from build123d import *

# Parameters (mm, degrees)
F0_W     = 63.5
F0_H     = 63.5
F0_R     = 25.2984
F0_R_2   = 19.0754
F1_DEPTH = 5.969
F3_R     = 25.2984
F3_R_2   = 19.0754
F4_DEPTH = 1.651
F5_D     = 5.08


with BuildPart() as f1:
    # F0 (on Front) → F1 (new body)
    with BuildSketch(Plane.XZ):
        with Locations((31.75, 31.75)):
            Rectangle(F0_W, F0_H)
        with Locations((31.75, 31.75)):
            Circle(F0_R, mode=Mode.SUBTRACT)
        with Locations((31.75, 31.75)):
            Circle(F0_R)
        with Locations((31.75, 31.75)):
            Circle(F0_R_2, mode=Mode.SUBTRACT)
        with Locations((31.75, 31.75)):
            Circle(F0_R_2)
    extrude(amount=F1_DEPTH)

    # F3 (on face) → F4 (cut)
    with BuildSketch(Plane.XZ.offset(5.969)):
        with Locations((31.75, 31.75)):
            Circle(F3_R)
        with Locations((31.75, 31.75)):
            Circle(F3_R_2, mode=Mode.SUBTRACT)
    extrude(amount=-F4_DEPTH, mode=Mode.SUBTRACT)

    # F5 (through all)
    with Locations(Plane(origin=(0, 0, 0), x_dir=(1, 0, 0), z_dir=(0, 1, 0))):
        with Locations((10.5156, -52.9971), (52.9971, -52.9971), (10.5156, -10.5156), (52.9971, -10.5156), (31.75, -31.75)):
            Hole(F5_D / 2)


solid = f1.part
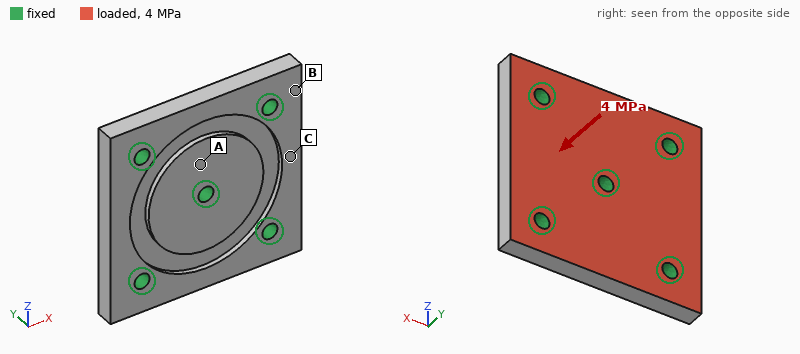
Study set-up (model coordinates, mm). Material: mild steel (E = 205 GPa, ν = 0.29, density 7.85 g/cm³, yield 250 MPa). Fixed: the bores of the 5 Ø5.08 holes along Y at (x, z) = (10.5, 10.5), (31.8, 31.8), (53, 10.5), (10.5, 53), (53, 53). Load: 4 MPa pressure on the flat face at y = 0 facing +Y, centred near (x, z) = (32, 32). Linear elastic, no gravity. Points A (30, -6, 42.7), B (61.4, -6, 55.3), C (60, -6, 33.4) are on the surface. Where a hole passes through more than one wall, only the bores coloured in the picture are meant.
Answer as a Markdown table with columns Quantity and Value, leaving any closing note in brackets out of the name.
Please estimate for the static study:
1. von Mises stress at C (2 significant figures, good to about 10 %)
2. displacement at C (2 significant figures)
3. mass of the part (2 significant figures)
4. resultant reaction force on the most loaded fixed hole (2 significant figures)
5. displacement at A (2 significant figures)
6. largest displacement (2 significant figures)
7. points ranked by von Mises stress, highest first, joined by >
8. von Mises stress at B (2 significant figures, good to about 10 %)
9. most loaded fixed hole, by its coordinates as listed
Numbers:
| Quantity | Value |
|---|---|
| von Mises stress at C | 46 MPa |
| displacement at C | 11 µm |
| mass of the part | 170 g |
| resultant reaction force on the most loaded fixed hole | 3.7 kN |
| displacement at A | 4.5 µm |
| largest displacement | 12 µm |
| points ranked by von Mises stress, highest first, joined by > | C > B > A |
| von Mises stress at B | 29 MPa |
| most loaded fixed hole, by its coordinates as listed | (31.8, 31.8) |
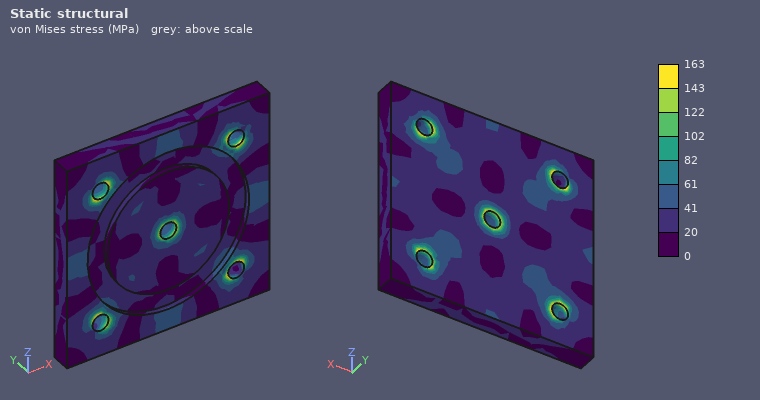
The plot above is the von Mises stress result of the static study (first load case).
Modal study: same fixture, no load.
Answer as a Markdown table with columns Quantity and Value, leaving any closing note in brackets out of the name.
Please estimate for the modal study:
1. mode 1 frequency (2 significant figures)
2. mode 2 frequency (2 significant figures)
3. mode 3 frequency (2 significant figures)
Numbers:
| Quantity | Value |
|---|---|
| mode 1 frequency | 16 kHz |
| mode 2 frequency | 17 kHz |
| mode 3 frequency | 17 kHz |
